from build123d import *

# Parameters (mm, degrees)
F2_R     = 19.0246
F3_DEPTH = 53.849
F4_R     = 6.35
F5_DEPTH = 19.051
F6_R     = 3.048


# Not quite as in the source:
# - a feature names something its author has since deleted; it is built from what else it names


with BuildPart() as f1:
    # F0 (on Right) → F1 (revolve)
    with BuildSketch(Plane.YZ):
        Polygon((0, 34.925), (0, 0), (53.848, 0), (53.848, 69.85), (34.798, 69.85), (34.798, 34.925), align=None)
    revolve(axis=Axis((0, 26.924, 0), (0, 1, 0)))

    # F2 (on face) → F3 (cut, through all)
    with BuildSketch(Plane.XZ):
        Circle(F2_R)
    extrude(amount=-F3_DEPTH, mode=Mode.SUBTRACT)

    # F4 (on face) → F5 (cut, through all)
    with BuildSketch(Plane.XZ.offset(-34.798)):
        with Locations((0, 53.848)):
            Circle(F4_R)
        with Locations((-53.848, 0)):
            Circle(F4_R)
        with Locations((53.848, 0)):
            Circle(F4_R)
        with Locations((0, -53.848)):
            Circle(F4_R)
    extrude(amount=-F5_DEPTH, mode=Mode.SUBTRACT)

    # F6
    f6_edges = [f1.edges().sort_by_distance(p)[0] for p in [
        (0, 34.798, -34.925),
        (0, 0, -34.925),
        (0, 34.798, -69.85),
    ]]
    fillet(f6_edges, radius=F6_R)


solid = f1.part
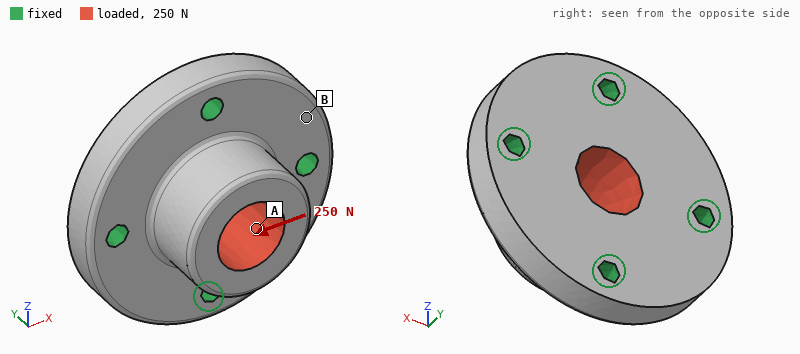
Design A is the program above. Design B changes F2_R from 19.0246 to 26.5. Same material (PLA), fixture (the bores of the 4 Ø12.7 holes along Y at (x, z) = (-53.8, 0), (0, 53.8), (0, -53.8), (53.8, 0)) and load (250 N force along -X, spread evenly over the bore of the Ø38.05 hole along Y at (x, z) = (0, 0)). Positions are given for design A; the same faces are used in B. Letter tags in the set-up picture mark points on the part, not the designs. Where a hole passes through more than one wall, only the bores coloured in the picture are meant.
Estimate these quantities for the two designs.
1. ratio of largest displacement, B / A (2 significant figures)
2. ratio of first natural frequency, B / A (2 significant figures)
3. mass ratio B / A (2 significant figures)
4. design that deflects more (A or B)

1.5
0.98
0.84
B
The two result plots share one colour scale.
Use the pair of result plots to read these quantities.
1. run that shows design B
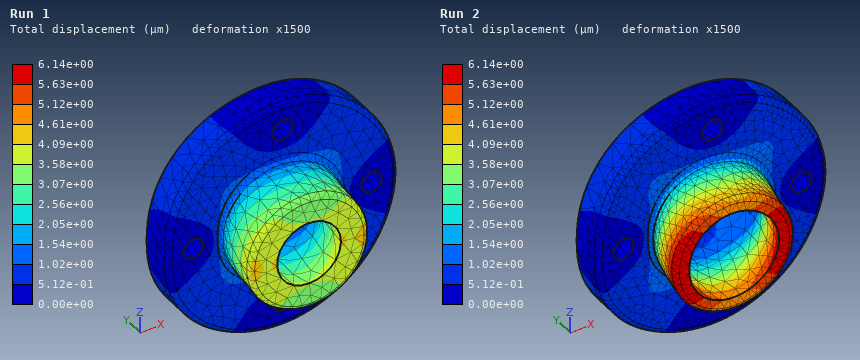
Run 2
